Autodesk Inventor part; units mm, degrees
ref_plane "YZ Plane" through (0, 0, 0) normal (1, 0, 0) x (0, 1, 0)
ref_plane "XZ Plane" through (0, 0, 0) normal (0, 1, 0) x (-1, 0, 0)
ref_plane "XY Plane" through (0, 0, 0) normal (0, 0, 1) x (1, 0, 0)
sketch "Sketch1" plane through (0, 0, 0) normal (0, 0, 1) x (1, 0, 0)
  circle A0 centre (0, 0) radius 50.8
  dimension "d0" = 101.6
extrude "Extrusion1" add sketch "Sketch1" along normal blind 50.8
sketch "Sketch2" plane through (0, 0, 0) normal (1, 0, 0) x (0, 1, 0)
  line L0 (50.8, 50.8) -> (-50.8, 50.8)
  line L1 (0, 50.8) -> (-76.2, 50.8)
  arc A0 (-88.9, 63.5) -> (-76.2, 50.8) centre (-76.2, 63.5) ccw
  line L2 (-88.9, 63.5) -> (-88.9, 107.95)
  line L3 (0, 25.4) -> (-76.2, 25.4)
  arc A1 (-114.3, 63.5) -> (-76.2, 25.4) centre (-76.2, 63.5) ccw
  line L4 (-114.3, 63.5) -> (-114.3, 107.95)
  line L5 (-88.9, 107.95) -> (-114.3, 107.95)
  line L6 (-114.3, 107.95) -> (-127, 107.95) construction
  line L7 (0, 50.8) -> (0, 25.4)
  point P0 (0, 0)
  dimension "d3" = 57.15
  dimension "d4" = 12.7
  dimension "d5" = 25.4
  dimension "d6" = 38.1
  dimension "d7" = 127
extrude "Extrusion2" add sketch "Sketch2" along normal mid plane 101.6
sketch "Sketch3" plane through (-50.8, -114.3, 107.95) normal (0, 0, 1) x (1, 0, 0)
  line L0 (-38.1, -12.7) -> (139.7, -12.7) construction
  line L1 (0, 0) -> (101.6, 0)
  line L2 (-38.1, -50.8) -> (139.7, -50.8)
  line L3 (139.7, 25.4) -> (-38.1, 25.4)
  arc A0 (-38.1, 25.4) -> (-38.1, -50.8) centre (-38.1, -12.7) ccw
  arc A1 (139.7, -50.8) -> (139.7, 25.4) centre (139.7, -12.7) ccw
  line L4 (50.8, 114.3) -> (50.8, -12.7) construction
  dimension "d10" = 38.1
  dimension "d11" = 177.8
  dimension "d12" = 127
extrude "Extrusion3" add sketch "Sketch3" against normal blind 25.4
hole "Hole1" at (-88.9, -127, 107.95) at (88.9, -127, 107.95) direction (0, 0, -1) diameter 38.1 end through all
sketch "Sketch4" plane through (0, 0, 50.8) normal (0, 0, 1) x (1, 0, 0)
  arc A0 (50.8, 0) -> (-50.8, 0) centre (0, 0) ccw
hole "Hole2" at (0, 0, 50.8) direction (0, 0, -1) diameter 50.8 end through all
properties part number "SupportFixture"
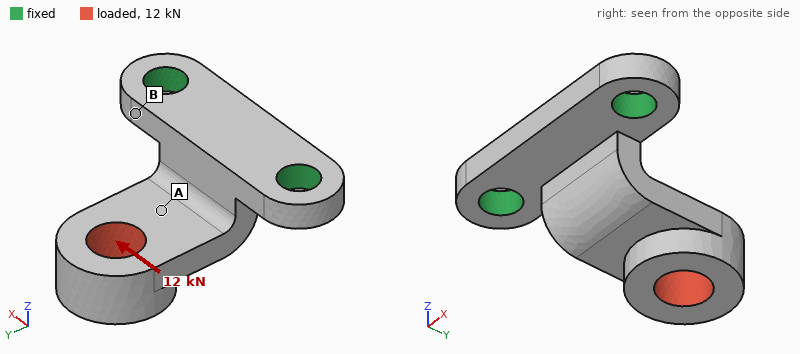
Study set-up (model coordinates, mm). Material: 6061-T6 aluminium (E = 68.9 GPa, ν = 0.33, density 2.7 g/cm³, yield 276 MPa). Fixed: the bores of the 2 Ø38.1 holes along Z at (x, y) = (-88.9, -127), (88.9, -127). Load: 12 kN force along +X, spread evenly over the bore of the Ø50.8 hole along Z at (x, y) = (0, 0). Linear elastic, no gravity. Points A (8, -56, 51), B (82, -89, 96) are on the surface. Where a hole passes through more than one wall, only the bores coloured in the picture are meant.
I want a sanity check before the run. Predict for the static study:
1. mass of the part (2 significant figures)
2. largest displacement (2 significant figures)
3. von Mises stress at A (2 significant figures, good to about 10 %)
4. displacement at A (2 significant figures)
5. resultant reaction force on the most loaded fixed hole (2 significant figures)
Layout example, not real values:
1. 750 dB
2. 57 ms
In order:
1. 2.6 kg
2. 0.46 mm
3. 17 MPa
4. 0.14 mm
5. 14 kN
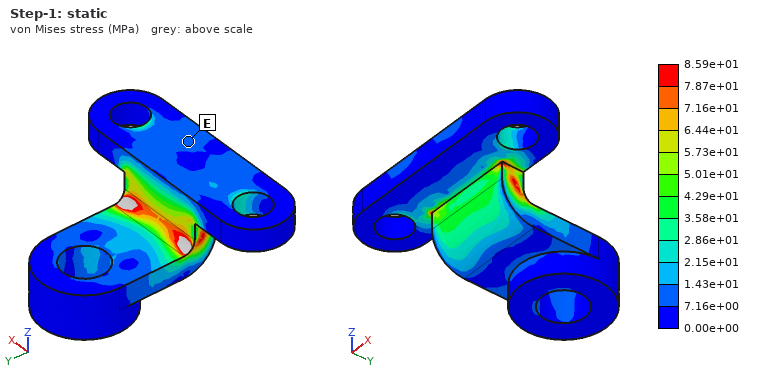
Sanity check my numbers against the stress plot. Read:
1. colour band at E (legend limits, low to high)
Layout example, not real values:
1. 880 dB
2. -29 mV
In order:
1. 7.16e+00 to 1.43e+01 MPa
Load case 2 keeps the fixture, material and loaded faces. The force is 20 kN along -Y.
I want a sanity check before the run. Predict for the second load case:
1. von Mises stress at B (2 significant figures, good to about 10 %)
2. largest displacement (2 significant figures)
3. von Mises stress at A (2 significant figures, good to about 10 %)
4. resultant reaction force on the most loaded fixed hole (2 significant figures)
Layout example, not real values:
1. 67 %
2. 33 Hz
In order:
1. 33 MPa
2. 1.6 mm
3. 17 MPa
4. 10 kN
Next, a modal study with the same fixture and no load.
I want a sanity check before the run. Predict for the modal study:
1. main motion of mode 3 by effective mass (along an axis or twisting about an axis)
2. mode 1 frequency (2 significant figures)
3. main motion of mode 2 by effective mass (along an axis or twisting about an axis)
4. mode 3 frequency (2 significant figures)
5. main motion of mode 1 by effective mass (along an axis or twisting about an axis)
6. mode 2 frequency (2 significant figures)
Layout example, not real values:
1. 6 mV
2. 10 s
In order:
1. along Y
2. 440 Hz
3. along X
4. 1900 Hz
5. along Z
6. 980 Hz
